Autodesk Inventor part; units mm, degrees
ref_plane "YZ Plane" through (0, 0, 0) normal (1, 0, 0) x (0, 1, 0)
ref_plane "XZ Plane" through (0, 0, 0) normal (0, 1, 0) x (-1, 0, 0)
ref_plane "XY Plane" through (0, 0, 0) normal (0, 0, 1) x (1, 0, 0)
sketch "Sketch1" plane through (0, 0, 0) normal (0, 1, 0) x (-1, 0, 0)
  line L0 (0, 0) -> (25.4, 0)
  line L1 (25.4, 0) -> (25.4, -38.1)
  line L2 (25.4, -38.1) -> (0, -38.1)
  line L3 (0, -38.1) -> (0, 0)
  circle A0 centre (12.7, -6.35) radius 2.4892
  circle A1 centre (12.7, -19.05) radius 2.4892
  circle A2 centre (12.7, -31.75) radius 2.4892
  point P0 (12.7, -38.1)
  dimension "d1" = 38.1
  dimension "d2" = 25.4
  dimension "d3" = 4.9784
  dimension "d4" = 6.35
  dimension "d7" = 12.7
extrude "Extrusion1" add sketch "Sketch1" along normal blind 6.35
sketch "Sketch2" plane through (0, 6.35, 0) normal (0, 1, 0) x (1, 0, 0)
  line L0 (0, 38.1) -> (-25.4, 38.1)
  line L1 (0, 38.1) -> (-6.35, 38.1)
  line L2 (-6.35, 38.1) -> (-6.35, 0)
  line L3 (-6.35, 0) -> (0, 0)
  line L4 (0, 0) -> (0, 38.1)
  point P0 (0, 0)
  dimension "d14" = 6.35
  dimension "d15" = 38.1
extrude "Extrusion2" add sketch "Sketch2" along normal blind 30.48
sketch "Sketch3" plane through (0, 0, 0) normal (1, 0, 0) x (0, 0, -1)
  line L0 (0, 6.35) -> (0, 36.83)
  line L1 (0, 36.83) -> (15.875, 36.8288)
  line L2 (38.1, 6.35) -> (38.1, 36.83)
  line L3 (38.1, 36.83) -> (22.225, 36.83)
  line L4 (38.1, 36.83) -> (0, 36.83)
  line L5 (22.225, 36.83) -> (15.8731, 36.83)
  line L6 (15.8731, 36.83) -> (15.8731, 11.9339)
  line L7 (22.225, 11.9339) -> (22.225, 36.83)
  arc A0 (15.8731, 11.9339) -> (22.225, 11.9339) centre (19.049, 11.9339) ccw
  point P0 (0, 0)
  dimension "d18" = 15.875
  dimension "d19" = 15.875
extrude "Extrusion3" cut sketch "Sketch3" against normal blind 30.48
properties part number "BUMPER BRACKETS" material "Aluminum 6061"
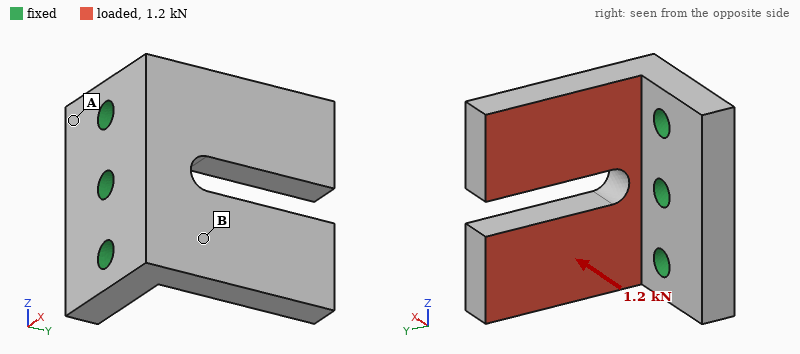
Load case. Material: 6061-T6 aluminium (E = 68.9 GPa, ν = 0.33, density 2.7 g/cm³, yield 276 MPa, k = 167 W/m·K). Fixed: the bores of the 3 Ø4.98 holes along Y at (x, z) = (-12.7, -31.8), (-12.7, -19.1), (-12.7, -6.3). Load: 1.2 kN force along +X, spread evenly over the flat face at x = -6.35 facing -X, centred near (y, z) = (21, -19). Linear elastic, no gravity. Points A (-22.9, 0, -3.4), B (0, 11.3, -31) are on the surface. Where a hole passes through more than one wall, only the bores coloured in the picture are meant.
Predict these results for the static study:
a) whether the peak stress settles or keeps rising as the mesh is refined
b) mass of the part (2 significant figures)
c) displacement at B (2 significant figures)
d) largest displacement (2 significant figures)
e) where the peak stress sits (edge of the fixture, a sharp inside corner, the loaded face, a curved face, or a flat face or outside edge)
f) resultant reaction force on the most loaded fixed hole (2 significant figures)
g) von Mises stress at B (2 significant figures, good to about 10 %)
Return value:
keeps rising
33 g
0.043 mm
0.21 mm
edge of the fixture
430 N
53 MPa
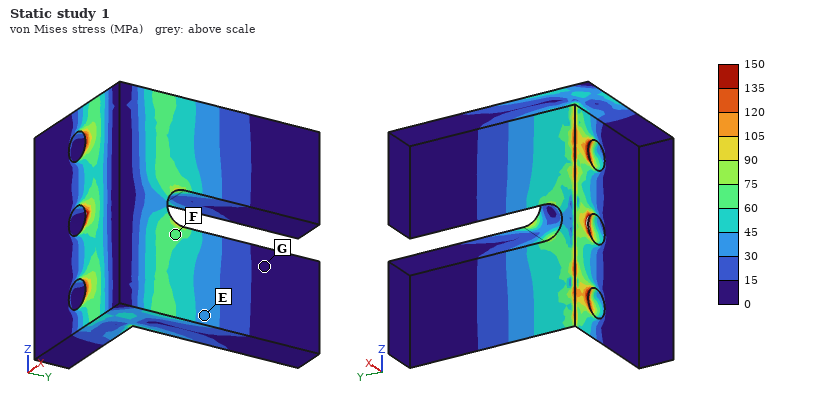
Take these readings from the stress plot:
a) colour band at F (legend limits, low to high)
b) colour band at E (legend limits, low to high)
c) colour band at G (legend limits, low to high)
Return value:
60 to 75 MPa
30 to 45 MPa
0 to 15 MPa
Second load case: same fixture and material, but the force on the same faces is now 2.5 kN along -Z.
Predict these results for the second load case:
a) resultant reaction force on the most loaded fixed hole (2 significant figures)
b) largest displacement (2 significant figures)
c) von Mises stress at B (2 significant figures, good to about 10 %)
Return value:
1.7 kN
0.12 mm
25 MPa
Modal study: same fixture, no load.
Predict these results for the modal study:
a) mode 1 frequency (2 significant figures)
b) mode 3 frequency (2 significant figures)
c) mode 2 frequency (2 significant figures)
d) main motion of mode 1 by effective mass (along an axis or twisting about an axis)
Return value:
3600 Hz
7700 Hz
4100 Hz
along X
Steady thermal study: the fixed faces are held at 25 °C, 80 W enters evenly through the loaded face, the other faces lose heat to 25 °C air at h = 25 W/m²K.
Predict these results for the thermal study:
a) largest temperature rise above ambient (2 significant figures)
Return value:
52 K
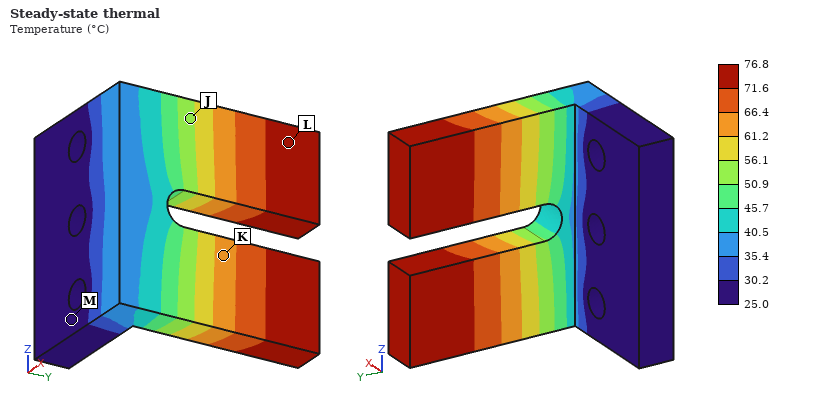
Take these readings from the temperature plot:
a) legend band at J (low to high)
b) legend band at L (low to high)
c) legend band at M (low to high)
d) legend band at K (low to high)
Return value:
50.9 to 56.1 °C
71.6 to 76.8 °C
25.0 to 30.2 °C
61.2 to 66.4 °C
